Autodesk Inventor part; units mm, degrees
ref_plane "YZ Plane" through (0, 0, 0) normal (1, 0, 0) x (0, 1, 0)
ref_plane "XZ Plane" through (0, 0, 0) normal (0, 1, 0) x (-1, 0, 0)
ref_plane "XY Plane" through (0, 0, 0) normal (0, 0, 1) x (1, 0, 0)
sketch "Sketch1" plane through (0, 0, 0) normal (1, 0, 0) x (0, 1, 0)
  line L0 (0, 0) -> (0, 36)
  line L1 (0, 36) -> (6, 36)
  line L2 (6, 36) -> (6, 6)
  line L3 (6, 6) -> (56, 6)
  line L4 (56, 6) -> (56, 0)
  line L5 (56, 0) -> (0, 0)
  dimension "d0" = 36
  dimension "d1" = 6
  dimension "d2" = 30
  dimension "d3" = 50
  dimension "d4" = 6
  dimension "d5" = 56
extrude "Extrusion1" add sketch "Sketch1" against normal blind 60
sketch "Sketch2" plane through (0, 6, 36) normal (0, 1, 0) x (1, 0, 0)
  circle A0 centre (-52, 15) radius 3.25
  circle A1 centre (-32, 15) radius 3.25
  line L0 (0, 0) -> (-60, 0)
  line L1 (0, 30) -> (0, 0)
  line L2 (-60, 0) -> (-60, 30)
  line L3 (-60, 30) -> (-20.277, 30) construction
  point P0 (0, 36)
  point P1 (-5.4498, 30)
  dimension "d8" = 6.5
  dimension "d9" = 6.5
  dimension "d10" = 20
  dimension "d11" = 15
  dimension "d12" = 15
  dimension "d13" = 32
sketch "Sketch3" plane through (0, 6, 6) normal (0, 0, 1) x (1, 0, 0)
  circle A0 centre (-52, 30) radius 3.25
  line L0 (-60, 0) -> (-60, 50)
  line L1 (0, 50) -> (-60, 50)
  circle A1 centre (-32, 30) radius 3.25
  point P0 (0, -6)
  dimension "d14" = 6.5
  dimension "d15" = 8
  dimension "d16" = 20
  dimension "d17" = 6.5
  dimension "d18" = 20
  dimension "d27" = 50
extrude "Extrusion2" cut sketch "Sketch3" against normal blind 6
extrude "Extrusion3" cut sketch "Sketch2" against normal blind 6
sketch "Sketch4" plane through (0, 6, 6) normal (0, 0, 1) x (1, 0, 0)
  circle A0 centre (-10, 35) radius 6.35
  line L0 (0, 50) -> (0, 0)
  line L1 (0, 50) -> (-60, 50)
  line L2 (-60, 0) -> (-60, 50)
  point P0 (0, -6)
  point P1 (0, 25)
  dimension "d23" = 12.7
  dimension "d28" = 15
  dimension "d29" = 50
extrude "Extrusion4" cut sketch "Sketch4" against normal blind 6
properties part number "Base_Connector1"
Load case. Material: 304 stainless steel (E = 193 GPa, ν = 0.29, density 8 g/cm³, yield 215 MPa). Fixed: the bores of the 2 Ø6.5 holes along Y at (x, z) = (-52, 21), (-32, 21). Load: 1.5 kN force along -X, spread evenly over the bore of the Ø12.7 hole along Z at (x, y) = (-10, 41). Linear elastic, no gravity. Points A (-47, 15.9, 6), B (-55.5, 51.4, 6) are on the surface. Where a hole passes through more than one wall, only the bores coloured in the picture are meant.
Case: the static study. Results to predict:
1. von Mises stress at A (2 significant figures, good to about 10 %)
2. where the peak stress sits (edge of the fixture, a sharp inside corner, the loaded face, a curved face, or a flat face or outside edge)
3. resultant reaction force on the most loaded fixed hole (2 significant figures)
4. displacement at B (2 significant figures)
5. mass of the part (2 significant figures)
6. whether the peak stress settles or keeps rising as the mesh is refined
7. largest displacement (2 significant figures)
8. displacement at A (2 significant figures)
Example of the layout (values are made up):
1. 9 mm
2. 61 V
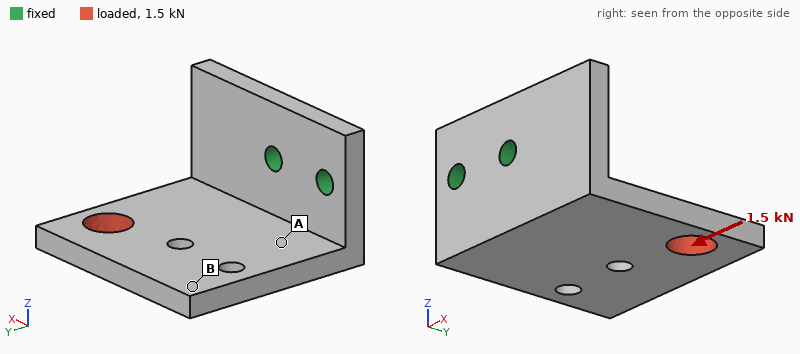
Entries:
1. 40 MPa
2. edge of the fixture
3. 2.4 kN
4. 0.087 mm
5. 240 g
6. keeps rising
7. 0.12 mm
8. 0.026 mm
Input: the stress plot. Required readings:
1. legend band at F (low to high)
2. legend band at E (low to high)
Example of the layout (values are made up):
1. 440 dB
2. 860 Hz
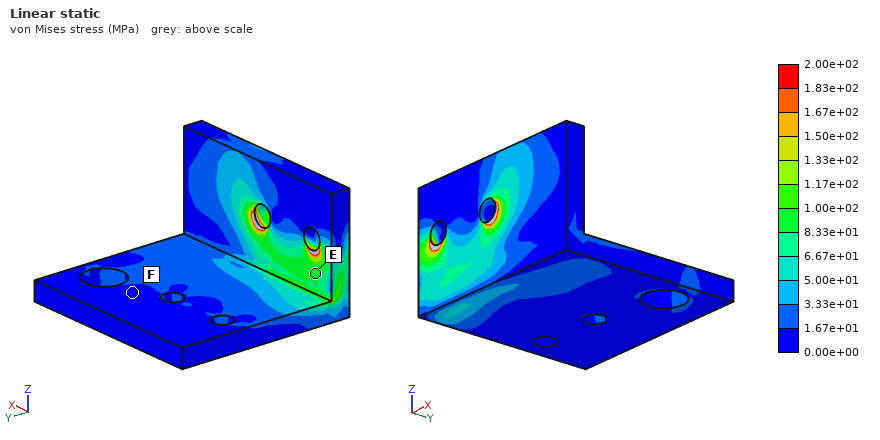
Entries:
1. 0.00e+00 to 1.67e+01 MPa
2. 8.33e+01 to 1.00e+02 MPa
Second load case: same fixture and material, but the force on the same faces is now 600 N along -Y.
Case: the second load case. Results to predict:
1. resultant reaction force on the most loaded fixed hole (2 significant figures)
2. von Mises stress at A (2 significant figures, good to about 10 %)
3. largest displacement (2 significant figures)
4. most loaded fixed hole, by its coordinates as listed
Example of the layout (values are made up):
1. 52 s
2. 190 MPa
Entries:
1. 940 N
2. 9.6 MPa
3. 57 µm
4. (-32, 21)
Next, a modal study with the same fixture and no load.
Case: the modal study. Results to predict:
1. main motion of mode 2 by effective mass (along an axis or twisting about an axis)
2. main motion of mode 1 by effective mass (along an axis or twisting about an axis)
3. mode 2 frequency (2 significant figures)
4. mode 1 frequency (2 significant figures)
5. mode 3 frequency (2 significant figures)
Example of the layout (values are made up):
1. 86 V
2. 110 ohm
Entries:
1. along X
2. along Z
3. 2100 Hz
4. 1100 Hz
5. 3400 Hz
